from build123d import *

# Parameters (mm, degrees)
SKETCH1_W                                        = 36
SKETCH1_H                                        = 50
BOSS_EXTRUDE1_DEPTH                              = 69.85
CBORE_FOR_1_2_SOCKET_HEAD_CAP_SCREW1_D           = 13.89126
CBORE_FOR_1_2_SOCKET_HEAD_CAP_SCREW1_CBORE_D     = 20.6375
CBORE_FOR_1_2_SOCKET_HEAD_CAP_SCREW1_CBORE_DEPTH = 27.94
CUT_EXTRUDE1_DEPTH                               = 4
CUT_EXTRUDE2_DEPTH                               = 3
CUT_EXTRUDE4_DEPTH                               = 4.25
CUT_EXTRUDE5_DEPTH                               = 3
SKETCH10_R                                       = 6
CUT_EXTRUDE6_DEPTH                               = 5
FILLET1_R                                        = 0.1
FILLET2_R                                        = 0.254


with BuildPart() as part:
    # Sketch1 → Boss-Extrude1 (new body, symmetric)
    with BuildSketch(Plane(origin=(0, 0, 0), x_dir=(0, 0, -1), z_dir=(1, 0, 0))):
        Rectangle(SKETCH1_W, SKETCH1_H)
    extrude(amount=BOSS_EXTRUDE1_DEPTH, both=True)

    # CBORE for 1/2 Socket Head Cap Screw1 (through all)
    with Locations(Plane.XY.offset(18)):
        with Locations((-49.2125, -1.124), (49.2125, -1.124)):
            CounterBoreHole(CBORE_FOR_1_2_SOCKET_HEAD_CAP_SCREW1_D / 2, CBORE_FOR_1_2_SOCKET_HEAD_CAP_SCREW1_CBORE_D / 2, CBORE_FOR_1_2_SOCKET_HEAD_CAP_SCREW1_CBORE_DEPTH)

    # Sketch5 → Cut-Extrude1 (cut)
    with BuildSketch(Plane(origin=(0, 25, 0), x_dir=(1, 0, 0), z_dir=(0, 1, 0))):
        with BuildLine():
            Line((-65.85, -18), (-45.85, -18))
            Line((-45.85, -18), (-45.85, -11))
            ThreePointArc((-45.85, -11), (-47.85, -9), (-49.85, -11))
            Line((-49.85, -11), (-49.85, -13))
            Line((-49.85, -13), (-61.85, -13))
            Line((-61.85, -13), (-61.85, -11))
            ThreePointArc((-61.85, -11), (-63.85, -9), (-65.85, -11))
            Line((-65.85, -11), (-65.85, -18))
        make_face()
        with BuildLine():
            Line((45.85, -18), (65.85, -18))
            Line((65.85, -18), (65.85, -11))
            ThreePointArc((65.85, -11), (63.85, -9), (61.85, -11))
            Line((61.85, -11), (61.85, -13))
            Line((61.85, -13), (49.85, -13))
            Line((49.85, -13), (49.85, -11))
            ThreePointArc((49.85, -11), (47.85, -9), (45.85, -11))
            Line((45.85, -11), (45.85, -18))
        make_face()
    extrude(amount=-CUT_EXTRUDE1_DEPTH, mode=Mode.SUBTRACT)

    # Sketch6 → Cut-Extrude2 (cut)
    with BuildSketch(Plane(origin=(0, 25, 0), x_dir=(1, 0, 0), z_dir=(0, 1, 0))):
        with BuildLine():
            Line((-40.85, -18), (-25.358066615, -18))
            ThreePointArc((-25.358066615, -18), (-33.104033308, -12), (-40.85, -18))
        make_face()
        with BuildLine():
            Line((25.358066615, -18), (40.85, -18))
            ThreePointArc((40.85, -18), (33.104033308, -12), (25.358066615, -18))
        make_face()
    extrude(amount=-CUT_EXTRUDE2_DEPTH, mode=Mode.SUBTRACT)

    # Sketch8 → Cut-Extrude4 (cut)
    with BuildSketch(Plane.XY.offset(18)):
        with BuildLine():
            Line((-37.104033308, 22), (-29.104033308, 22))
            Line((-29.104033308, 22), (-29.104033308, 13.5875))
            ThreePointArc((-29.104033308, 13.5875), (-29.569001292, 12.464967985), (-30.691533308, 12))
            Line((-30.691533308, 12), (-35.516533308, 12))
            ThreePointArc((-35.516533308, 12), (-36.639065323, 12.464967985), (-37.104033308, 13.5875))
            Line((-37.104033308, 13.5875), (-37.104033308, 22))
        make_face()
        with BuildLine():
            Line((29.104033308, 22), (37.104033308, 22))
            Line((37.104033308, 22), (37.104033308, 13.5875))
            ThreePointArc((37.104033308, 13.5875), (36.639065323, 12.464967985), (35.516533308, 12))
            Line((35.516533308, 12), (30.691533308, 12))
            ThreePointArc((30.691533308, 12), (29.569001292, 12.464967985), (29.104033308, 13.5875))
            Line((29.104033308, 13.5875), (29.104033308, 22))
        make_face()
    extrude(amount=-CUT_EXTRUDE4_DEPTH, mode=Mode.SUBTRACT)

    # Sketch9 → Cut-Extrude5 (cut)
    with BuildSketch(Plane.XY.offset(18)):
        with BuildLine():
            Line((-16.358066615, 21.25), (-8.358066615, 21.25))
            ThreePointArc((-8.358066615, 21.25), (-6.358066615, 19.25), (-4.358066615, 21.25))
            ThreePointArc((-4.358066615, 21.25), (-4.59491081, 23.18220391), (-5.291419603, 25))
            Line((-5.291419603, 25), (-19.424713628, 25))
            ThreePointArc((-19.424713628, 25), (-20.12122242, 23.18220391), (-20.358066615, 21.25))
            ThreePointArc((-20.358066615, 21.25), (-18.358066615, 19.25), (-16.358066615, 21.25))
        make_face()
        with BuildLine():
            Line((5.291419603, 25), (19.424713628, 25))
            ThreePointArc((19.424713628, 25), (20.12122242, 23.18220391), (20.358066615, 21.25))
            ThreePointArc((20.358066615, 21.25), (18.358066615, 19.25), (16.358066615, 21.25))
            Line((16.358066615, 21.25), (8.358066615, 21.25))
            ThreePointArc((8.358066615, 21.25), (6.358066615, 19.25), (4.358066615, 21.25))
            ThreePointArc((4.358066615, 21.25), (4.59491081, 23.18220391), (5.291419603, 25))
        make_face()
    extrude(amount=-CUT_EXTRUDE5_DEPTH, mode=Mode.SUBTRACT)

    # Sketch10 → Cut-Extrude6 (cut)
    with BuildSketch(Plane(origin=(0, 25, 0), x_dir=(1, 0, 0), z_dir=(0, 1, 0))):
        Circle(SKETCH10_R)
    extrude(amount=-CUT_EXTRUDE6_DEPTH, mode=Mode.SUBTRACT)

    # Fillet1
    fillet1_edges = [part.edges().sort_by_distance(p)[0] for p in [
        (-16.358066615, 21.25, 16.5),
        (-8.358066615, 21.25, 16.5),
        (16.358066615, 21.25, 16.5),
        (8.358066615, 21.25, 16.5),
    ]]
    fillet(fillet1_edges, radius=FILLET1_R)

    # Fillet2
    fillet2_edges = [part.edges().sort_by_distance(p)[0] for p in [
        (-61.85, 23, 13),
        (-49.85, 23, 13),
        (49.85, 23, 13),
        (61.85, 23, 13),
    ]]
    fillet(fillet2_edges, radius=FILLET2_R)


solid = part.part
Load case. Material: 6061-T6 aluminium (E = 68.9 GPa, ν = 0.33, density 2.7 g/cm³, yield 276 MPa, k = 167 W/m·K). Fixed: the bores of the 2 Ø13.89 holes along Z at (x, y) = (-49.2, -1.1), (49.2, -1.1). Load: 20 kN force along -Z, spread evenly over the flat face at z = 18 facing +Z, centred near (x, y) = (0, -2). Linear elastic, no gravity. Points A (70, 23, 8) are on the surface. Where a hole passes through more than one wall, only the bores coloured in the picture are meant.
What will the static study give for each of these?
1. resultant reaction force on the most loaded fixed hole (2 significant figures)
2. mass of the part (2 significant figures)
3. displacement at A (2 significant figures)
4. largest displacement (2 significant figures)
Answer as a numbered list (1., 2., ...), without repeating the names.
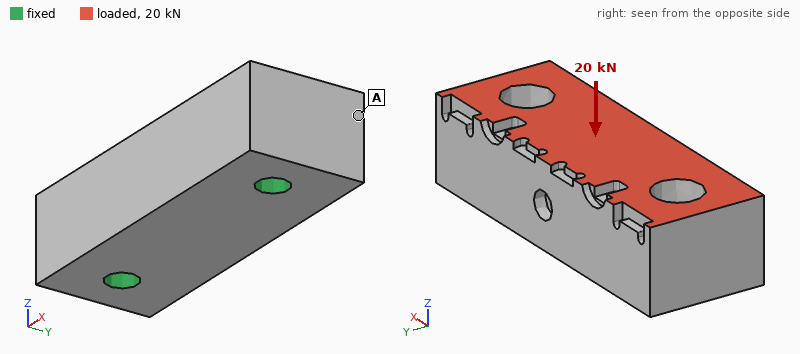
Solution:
1. 11 kN
2. 610 g
3. 3.9 µm
4. 21 µm
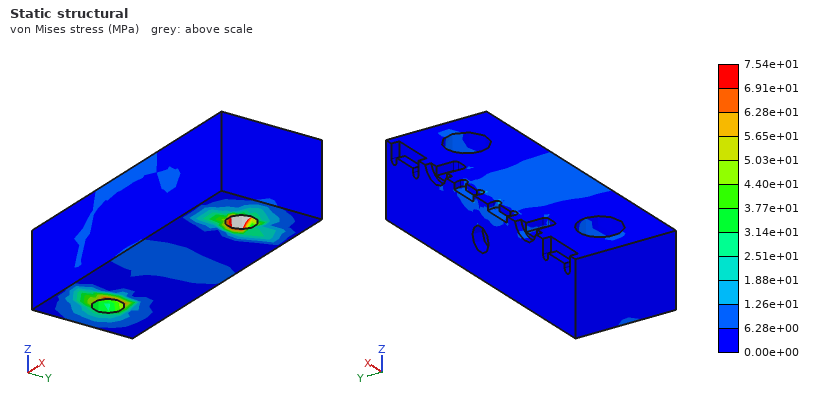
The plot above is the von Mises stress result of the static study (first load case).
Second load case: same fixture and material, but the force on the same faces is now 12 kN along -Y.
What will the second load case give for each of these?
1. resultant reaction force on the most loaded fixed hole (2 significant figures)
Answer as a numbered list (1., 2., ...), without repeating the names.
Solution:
1. 6.0 kN
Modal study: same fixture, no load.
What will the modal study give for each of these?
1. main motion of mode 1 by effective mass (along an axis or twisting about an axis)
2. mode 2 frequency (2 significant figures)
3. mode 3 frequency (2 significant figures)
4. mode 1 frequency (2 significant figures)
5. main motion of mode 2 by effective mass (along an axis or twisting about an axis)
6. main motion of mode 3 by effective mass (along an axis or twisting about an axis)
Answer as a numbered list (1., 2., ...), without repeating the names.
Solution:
1. along Y
2. 7600 Hz
3. 8200 Hz
4. 3400 Hz
5. along Z
6. twisting about Z
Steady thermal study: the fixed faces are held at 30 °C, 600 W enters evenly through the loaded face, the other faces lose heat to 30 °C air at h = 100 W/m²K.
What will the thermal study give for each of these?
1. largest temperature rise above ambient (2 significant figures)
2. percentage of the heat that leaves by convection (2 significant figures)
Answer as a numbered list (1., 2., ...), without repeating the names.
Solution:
1. 53 K
2. 14 %
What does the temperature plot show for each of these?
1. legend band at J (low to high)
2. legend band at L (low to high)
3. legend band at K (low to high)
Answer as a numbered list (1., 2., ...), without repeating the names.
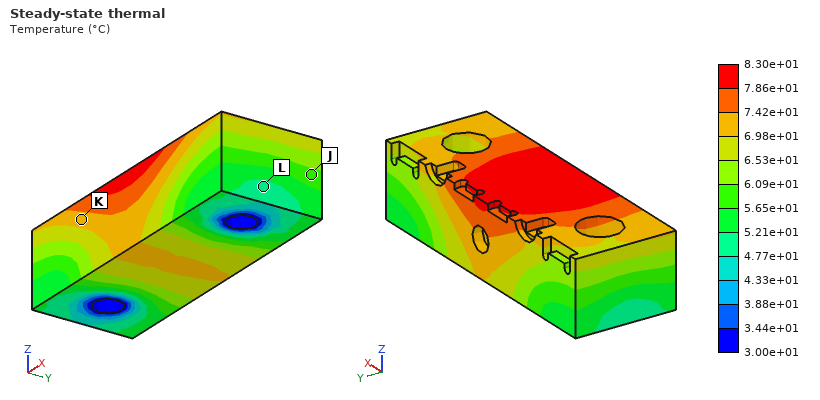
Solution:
1. 5.65e+01 to 6.09e+01 °C
2. 4.77e+01 to 5.21e+01 °C
3. 6.98e+01 to 7.42e+01 °C
